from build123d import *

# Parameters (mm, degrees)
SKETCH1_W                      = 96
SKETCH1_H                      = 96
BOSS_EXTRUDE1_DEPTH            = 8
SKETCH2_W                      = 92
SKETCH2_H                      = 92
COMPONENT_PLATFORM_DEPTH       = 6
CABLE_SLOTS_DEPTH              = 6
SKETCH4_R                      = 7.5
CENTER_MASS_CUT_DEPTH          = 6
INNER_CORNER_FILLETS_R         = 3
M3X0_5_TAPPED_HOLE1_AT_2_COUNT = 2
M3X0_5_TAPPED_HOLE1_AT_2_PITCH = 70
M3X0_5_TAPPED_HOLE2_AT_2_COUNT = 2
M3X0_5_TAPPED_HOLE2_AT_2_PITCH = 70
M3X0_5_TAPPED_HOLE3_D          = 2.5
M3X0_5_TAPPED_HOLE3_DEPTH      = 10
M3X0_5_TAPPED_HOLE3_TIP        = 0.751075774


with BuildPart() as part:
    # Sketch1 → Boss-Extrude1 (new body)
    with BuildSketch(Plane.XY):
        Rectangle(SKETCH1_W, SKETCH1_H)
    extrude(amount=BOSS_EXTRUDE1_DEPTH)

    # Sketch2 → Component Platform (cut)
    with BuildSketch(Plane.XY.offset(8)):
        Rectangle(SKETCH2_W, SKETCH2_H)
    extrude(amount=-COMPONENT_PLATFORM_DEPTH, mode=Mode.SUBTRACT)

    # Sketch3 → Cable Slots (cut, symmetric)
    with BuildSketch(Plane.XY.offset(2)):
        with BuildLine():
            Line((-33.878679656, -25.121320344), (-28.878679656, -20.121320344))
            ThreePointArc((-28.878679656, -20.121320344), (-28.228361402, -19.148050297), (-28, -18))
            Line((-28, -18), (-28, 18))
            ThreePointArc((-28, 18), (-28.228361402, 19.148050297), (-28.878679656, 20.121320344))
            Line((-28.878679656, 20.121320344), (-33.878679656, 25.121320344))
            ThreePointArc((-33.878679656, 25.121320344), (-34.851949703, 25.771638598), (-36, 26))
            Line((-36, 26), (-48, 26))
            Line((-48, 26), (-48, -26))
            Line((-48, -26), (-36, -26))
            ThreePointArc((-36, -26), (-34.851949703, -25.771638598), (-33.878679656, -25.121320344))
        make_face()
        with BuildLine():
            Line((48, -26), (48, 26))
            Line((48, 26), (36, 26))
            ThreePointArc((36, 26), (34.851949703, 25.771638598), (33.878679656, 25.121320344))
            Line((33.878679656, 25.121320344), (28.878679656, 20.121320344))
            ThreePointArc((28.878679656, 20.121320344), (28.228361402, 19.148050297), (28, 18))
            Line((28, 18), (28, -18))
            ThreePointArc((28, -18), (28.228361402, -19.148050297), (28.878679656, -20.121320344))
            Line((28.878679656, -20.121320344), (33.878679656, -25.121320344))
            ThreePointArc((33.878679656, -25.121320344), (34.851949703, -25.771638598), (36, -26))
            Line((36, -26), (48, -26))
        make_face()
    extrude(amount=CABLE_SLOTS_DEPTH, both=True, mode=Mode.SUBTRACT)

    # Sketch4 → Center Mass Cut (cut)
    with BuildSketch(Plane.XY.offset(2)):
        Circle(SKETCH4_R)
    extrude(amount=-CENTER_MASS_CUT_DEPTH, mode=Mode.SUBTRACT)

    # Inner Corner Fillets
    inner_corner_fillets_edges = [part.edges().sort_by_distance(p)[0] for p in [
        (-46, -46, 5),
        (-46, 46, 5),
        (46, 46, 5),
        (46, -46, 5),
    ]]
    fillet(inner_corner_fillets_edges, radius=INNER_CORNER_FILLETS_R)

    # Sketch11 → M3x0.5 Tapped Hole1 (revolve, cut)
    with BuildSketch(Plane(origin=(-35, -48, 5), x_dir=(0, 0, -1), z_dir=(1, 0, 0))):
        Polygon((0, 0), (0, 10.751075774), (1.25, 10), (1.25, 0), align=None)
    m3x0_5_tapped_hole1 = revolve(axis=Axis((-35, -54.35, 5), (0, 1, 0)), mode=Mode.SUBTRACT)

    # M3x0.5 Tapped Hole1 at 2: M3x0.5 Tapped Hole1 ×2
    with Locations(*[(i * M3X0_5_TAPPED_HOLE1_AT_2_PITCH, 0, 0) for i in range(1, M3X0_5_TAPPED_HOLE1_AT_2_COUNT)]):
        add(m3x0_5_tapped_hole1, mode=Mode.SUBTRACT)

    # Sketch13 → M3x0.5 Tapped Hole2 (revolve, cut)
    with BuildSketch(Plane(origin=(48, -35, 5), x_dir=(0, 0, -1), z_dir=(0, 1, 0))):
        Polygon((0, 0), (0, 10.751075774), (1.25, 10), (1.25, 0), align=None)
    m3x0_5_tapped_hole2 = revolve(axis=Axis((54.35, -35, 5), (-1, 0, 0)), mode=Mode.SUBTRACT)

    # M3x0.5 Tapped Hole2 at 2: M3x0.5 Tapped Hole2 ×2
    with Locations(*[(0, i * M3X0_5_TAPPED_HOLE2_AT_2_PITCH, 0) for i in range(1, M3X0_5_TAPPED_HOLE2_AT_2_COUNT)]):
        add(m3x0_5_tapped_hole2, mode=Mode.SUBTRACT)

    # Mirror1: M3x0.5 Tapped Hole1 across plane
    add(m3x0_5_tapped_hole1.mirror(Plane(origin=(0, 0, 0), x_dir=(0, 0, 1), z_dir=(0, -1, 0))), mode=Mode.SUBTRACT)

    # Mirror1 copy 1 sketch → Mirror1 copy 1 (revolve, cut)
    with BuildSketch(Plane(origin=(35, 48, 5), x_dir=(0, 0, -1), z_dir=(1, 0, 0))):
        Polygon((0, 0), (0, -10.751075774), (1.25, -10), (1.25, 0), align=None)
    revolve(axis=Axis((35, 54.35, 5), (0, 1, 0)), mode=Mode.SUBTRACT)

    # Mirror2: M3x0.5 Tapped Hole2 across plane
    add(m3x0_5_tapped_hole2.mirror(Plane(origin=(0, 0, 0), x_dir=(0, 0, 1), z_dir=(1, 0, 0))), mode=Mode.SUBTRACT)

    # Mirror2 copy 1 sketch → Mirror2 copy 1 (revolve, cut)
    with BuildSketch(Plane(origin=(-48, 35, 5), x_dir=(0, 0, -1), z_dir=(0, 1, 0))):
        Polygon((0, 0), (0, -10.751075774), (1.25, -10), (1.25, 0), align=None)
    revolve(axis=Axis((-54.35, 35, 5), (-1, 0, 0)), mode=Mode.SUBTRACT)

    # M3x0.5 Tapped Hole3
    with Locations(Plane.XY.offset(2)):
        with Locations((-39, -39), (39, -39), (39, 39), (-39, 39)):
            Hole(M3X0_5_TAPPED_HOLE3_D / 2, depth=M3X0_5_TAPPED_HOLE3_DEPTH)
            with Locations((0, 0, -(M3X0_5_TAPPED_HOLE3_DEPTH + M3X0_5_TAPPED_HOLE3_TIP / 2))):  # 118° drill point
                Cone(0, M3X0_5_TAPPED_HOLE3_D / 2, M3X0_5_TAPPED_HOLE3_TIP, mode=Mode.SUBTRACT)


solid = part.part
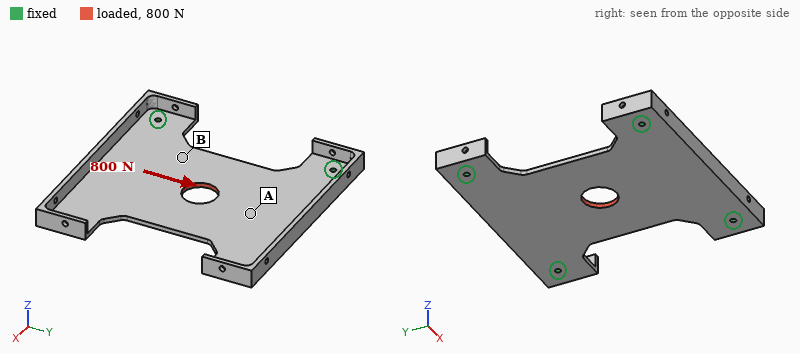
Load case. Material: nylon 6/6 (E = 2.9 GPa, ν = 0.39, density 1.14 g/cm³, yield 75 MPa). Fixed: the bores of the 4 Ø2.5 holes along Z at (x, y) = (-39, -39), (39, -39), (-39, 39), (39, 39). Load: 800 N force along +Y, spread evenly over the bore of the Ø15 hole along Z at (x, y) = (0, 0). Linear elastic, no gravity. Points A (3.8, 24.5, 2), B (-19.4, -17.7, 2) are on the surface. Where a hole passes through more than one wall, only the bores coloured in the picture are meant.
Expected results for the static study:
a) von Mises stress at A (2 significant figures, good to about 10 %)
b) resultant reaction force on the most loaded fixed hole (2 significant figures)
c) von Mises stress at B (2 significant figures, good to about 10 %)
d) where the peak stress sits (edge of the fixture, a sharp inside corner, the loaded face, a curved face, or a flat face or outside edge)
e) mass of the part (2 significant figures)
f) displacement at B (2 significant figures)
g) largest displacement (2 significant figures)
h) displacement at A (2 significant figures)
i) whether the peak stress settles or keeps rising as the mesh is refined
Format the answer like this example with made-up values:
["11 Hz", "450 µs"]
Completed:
["2.6 MPa", "230 N", "7.2 MPa", "edge of the fixture", "20 g", "0.13 mm", "0.25 mm", "0.17 mm", "keeps rising"]
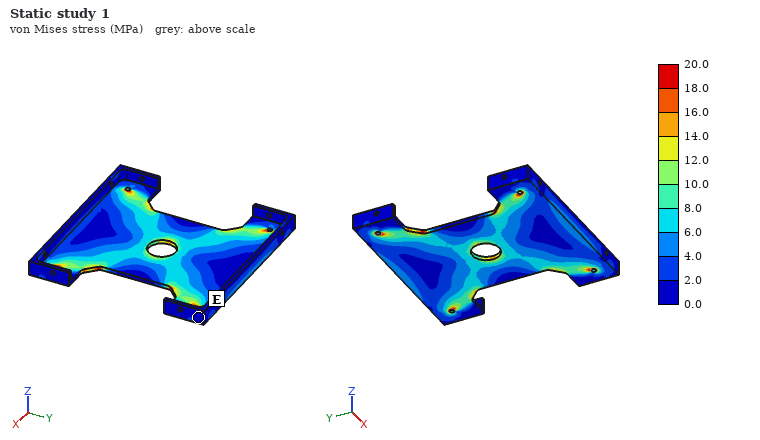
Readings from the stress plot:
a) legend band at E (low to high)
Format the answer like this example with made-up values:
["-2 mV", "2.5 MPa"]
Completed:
["0.0 to 2.0 MPa"]
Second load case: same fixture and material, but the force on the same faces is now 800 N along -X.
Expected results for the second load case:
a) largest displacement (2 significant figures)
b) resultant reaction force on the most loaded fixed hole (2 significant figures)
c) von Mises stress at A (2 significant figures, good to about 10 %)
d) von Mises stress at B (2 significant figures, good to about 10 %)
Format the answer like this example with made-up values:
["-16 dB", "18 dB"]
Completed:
["0.17 mm", "230 N", "4.7 MPa", "7.0 MPa"]
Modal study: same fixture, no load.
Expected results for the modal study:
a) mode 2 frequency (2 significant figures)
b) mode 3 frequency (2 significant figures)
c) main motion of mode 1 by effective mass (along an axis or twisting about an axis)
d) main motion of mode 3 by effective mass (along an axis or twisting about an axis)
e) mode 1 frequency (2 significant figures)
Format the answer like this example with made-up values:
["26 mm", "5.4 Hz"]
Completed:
["740 Hz", "820 Hz", "along Z", "twisting about X", "370 Hz"]
